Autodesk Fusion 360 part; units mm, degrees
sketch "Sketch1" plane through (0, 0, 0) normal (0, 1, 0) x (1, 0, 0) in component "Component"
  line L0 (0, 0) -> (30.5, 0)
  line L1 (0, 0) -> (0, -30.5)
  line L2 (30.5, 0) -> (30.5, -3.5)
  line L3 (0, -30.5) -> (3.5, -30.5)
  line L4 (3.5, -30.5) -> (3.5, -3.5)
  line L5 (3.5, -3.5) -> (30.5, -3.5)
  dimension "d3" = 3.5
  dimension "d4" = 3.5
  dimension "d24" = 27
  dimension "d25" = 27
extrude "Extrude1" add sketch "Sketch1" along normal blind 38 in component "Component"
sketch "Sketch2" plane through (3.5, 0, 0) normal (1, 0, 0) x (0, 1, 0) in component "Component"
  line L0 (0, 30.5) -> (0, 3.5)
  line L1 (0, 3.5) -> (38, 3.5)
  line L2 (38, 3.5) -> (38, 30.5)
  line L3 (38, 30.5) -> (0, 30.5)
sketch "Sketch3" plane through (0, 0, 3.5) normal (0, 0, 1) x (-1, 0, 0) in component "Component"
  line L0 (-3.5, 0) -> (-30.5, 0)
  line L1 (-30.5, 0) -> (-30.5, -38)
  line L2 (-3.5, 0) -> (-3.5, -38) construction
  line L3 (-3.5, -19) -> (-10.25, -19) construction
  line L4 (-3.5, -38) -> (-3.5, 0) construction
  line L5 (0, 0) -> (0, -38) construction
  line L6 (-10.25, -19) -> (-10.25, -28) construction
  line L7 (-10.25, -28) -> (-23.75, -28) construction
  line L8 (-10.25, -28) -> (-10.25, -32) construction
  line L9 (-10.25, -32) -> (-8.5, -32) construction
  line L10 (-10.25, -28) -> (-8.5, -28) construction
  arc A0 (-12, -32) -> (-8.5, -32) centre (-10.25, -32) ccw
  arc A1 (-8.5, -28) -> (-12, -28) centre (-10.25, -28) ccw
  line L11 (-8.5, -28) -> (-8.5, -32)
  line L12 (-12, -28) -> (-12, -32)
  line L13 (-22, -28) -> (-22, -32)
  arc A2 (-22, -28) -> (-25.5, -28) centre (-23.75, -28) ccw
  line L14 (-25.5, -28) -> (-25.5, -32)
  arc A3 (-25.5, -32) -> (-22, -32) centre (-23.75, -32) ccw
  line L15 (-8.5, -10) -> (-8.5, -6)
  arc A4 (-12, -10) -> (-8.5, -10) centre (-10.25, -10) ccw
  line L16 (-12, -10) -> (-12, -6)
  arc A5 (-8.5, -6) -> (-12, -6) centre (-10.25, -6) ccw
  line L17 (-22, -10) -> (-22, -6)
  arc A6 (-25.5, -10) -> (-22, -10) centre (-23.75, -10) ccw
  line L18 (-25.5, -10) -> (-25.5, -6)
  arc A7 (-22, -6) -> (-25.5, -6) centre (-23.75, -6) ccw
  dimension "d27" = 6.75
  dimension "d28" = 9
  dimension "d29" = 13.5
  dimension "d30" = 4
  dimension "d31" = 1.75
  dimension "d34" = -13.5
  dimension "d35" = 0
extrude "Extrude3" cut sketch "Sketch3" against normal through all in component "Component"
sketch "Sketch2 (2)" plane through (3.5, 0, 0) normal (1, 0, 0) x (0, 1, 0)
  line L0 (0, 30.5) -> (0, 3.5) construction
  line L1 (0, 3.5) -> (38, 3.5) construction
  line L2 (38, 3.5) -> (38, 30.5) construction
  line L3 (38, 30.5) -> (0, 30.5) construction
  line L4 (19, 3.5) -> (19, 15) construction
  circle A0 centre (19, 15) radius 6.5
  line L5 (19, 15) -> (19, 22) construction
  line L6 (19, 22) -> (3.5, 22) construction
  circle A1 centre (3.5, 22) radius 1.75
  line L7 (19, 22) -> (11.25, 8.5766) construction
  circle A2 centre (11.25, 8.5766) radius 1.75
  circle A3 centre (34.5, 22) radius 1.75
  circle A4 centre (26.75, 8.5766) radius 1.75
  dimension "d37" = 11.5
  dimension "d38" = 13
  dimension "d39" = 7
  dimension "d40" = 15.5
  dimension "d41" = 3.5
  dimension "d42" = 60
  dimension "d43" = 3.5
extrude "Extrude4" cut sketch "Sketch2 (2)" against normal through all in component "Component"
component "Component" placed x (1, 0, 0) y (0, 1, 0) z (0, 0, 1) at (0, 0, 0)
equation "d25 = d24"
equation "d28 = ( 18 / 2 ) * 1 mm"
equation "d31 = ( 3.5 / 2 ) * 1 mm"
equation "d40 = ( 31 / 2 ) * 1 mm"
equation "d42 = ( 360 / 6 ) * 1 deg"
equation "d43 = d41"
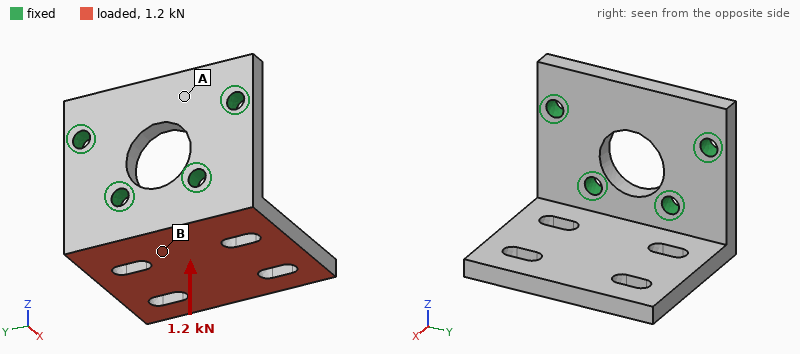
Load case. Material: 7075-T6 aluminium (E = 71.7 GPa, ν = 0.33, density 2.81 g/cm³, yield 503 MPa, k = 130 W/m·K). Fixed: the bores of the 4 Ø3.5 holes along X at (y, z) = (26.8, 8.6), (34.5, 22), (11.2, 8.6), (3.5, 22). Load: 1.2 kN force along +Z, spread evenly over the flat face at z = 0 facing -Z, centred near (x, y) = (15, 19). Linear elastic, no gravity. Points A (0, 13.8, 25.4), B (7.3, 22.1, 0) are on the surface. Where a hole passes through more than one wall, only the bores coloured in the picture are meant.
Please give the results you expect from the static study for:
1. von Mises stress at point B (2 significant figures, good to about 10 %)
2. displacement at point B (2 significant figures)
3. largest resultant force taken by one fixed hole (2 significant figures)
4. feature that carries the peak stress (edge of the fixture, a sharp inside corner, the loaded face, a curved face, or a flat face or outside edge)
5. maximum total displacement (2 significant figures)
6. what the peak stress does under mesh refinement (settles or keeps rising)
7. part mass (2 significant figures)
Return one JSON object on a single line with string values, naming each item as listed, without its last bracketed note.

{"von Mises stress at point B": "160 MPa", "displacement at point B": "0.11 mm", "largest resultant force taken by one fixed hole": "560 N", "feature that carries the peak stress": "edge of the fixture", "maximum total displacement": "0.69 mm", "what the peak stress does under mesh refinement": "keeps rising", "part mass": "19 g"}
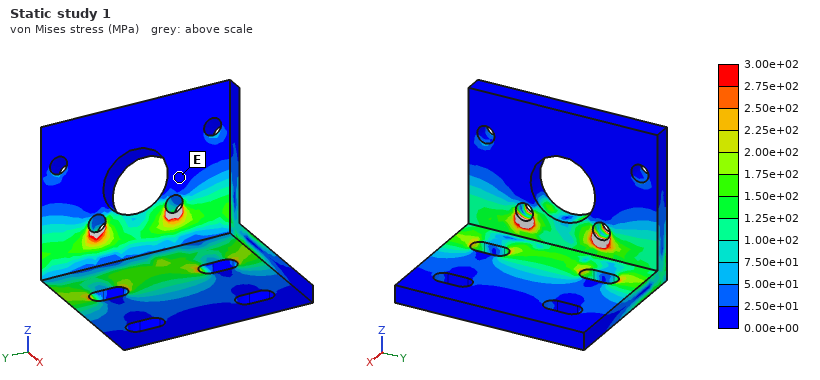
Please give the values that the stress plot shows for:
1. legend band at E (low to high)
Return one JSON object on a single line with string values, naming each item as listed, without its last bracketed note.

{"legend band at E": "0.00e+00 to 2.50e+01 MPa"}
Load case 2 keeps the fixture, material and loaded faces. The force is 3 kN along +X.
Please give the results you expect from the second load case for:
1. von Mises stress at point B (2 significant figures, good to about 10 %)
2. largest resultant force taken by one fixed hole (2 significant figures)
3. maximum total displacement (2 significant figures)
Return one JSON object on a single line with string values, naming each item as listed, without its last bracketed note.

{"von Mises stress at point B": "82 MPa", "largest resultant force taken by one fixed hole": "1.7 kN", "maximum total displacement": "0.50 mm"}
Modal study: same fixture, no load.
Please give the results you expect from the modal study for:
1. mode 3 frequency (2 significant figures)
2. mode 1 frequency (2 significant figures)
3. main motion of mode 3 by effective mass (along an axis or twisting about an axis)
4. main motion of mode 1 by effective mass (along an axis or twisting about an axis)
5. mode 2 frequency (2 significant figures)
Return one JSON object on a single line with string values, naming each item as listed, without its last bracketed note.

{"mode 3 frequency": "7700 Hz", "mode 1 frequency": "2500 Hz", "main motion of mode 3 by effective mass": "along Y", "main motion of mode 1 by effective mass": "along Z", "mode 2 frequency": "5400 Hz"}
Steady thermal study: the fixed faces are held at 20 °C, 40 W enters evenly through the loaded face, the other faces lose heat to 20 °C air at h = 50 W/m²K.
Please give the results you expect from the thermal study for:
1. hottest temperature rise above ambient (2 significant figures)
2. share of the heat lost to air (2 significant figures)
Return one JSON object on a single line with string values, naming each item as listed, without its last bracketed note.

{"hottest temperature rise above ambient": "50 K", "share of the heat lost to air": "8.6 %"}
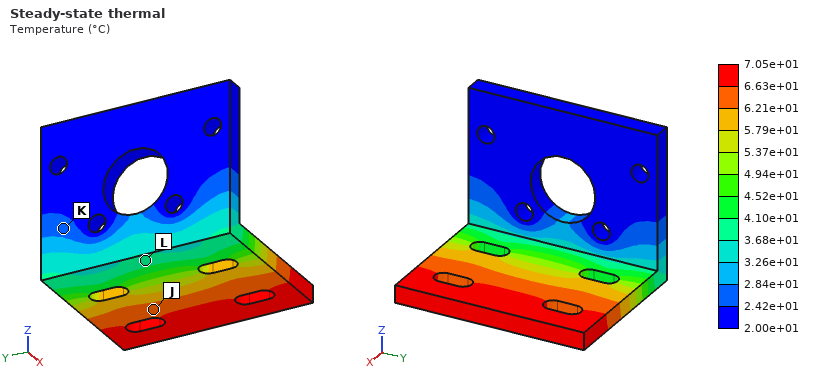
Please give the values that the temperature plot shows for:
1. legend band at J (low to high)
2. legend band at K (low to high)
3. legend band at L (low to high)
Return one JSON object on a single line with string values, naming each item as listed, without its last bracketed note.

{"legend band at J": "6.21e+01 to 6.63e+01 °C", "legend band at K": "2.42e+01 to 2.84e+01 °C", "legend band at L": "3.68e+01 to 4.10e+01 °C"}
